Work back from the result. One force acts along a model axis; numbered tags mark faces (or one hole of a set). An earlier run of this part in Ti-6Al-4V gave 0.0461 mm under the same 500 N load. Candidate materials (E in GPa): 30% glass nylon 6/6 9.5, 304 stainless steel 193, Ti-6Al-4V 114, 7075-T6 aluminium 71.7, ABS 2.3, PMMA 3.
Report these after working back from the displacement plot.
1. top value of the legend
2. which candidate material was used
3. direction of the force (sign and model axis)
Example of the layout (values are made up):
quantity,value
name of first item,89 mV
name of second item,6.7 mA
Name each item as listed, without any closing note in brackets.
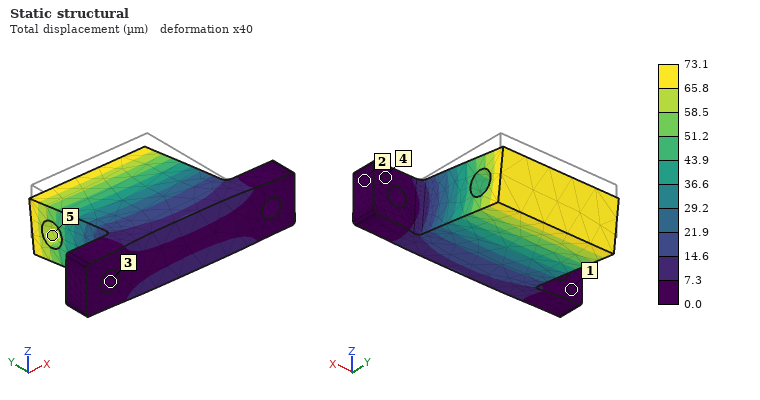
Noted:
quantity,value
top value of the legend,73.1 µm
which candidate material was used,7075-T6 aluminium
direction of the force,-Z
